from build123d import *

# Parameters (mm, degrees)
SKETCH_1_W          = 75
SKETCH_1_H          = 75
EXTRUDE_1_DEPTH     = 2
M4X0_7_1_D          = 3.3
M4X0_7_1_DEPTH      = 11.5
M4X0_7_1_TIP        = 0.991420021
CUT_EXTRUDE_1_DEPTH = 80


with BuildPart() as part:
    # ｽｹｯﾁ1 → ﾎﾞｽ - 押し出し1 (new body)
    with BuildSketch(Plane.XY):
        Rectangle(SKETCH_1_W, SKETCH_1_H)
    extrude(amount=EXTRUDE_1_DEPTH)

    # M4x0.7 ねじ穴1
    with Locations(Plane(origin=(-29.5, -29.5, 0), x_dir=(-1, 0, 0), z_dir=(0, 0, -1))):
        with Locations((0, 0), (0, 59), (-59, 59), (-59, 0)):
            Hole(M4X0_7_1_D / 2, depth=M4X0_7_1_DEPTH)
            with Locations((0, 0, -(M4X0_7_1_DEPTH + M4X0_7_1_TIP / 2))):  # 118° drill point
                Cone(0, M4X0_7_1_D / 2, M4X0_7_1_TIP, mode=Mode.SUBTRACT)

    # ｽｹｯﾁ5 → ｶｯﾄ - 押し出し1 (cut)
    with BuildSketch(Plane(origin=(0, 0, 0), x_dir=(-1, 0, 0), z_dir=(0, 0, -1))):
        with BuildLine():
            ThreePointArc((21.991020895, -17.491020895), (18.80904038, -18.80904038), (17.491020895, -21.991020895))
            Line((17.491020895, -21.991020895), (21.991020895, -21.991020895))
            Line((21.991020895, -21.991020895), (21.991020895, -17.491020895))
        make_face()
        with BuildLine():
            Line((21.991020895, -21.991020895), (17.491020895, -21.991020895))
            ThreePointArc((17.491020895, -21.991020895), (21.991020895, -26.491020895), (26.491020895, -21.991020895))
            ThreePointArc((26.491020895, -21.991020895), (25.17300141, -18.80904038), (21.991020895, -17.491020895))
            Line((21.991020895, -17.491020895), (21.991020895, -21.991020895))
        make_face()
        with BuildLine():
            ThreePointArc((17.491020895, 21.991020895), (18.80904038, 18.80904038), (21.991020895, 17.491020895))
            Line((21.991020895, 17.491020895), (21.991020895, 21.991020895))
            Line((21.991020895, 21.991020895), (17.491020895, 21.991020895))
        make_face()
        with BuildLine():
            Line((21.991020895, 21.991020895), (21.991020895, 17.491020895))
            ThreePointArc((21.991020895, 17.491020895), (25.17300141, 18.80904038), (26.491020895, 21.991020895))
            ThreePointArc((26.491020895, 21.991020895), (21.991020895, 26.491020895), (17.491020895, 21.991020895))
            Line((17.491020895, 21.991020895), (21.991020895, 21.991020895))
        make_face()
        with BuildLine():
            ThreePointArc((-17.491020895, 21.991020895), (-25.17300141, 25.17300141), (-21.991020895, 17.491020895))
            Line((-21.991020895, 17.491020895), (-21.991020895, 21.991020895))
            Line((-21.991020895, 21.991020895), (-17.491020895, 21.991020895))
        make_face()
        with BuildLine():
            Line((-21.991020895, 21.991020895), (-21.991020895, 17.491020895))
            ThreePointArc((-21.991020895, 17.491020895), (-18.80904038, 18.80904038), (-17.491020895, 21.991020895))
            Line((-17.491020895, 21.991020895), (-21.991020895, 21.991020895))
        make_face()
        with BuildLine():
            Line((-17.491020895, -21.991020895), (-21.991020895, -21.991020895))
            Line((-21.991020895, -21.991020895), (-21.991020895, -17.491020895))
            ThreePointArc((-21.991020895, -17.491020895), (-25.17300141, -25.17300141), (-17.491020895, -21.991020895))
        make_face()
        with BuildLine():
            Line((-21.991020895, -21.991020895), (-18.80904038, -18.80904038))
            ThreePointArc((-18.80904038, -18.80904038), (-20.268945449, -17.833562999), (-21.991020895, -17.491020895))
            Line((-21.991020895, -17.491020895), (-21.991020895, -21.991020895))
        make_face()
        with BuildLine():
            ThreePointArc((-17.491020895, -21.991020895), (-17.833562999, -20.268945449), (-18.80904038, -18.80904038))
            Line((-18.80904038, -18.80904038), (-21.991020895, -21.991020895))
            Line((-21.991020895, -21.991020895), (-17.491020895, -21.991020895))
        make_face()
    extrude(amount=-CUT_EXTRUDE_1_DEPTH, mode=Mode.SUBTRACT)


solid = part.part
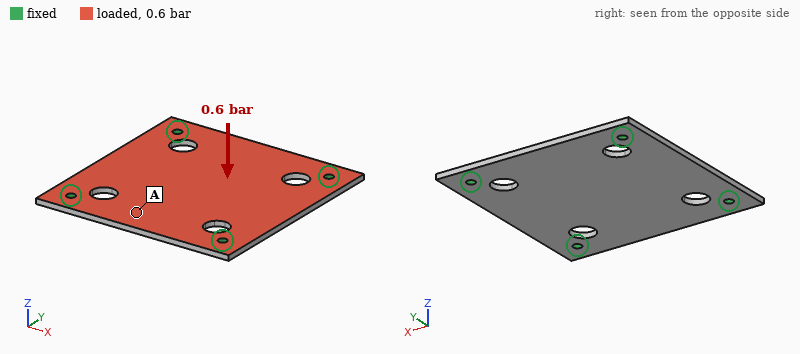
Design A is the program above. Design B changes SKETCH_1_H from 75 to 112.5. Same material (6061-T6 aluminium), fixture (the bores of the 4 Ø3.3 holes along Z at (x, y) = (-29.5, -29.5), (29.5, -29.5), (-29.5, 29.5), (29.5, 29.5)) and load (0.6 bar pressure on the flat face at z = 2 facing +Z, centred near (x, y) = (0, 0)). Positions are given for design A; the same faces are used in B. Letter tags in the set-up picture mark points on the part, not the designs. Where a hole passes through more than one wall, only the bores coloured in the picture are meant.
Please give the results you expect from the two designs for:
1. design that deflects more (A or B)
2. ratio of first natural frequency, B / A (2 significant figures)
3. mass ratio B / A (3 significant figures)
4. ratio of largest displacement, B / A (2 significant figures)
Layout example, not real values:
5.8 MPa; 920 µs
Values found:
B; 0.84; 1.53; 1.5
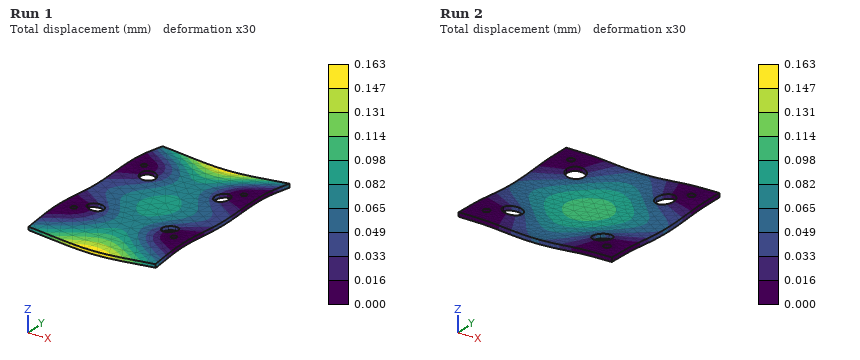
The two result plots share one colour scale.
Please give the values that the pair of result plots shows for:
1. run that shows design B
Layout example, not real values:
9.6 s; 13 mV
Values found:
Run 1
